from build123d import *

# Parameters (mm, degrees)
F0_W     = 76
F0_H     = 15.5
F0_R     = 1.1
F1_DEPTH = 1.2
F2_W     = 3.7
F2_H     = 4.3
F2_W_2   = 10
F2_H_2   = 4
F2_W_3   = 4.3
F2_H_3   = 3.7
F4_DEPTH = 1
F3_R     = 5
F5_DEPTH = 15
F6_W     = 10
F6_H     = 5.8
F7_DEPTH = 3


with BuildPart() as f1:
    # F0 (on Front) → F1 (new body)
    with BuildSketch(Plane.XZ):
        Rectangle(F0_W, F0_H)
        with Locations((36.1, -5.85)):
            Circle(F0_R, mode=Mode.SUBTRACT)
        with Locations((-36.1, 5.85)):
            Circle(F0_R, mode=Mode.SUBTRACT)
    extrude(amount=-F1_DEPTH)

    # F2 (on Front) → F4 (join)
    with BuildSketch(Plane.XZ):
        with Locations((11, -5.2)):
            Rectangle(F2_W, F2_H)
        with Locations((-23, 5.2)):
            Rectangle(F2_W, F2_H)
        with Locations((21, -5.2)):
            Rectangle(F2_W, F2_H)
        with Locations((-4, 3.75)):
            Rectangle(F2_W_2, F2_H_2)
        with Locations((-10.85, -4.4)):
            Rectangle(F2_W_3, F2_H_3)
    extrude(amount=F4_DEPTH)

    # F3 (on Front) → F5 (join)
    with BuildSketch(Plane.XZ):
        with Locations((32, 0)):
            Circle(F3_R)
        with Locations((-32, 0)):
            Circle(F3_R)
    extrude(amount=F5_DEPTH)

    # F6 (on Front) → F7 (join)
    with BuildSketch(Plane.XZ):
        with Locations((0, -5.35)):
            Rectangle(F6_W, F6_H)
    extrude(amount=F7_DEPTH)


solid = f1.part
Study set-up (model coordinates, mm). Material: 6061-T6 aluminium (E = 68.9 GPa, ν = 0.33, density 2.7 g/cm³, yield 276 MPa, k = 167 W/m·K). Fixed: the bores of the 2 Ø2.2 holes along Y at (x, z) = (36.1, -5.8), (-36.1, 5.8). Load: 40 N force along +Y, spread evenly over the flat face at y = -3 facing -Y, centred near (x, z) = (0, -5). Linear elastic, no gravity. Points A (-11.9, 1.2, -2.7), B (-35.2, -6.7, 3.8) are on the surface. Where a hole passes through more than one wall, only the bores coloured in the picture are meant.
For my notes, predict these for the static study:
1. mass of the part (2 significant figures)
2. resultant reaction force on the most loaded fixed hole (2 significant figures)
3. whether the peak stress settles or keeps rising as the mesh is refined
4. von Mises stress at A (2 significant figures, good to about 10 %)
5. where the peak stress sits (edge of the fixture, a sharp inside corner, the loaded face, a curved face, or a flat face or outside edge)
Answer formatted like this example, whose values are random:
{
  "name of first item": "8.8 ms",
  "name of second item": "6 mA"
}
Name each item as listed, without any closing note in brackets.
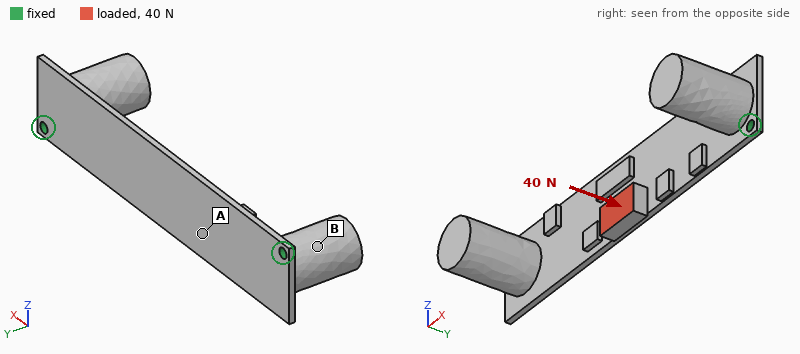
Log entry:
{
  "mass of the part": "11 g",
  "resultant reaction force on the most loaded fixed hole": "21 N",
  "whether the peak stress settles or keeps rising as the mesh is refined": "keeps rising",
  "von Mises stress at A": "29 MPa",
  "where the peak stress sits": "edge of the fixture"
}
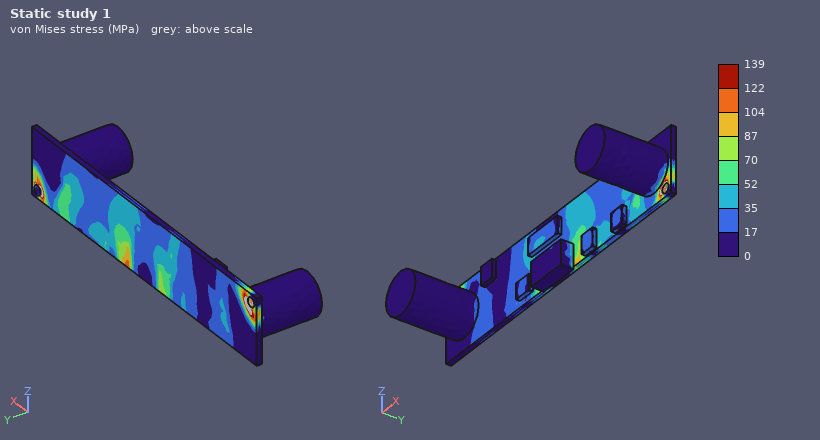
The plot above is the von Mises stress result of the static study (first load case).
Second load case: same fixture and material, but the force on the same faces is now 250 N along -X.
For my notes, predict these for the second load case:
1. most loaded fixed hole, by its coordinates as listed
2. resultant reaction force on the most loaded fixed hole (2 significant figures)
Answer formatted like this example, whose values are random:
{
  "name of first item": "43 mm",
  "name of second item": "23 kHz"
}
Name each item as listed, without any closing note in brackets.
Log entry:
{
  "most loaded fixed hole, by its coordinates as listed": "(-36.1, 5.8)",
  "resultant reaction force on the most loaded fixed hole": "150 N"
}
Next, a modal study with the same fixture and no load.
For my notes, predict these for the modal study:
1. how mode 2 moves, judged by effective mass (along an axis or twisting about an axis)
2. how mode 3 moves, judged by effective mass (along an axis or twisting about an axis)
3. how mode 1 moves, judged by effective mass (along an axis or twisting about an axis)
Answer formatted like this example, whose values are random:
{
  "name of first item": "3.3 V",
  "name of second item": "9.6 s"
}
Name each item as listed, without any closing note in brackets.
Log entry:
{
  "how mode 2 moves, judged by effective mass": "along Z",
  "how mode 3 moves, judged by effective mass": "twisting about Y",
  "how mode 1 moves, judged by effective mass": "along Y"
}
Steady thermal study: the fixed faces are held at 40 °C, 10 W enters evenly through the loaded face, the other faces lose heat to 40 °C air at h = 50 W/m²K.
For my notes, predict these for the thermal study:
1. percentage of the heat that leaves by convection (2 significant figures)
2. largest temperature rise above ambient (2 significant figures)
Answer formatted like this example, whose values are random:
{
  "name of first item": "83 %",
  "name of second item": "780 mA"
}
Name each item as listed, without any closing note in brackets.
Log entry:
{
  "percentage of the heat that leaves by convection": "34 %",
  "largest temperature rise above ambient": "50 K"
}
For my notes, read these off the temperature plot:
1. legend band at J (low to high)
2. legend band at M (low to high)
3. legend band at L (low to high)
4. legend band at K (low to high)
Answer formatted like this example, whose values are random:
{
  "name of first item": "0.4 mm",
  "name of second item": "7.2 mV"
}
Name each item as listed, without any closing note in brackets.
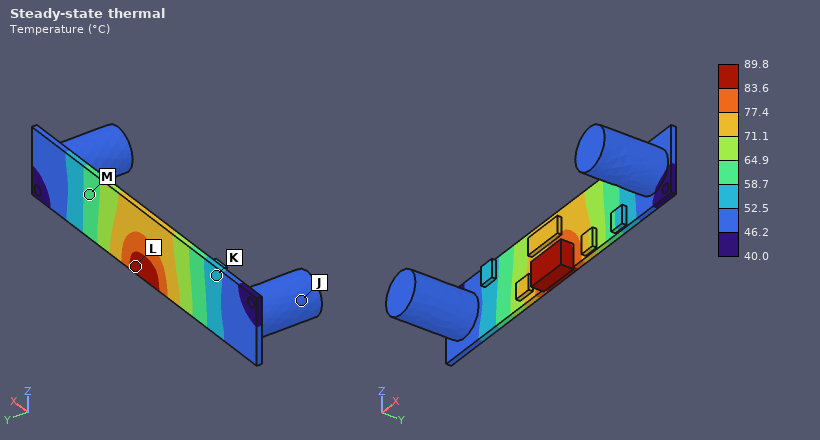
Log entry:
{
  "legend band at J": "46.2 to 52.5 °C",
  "legend band at M": "58.7 to 64.9 °C",
  "legend band at L": "83.6 to 89.8 °C",
  "legend band at K": "52.5 to 58.7 °C"
}
